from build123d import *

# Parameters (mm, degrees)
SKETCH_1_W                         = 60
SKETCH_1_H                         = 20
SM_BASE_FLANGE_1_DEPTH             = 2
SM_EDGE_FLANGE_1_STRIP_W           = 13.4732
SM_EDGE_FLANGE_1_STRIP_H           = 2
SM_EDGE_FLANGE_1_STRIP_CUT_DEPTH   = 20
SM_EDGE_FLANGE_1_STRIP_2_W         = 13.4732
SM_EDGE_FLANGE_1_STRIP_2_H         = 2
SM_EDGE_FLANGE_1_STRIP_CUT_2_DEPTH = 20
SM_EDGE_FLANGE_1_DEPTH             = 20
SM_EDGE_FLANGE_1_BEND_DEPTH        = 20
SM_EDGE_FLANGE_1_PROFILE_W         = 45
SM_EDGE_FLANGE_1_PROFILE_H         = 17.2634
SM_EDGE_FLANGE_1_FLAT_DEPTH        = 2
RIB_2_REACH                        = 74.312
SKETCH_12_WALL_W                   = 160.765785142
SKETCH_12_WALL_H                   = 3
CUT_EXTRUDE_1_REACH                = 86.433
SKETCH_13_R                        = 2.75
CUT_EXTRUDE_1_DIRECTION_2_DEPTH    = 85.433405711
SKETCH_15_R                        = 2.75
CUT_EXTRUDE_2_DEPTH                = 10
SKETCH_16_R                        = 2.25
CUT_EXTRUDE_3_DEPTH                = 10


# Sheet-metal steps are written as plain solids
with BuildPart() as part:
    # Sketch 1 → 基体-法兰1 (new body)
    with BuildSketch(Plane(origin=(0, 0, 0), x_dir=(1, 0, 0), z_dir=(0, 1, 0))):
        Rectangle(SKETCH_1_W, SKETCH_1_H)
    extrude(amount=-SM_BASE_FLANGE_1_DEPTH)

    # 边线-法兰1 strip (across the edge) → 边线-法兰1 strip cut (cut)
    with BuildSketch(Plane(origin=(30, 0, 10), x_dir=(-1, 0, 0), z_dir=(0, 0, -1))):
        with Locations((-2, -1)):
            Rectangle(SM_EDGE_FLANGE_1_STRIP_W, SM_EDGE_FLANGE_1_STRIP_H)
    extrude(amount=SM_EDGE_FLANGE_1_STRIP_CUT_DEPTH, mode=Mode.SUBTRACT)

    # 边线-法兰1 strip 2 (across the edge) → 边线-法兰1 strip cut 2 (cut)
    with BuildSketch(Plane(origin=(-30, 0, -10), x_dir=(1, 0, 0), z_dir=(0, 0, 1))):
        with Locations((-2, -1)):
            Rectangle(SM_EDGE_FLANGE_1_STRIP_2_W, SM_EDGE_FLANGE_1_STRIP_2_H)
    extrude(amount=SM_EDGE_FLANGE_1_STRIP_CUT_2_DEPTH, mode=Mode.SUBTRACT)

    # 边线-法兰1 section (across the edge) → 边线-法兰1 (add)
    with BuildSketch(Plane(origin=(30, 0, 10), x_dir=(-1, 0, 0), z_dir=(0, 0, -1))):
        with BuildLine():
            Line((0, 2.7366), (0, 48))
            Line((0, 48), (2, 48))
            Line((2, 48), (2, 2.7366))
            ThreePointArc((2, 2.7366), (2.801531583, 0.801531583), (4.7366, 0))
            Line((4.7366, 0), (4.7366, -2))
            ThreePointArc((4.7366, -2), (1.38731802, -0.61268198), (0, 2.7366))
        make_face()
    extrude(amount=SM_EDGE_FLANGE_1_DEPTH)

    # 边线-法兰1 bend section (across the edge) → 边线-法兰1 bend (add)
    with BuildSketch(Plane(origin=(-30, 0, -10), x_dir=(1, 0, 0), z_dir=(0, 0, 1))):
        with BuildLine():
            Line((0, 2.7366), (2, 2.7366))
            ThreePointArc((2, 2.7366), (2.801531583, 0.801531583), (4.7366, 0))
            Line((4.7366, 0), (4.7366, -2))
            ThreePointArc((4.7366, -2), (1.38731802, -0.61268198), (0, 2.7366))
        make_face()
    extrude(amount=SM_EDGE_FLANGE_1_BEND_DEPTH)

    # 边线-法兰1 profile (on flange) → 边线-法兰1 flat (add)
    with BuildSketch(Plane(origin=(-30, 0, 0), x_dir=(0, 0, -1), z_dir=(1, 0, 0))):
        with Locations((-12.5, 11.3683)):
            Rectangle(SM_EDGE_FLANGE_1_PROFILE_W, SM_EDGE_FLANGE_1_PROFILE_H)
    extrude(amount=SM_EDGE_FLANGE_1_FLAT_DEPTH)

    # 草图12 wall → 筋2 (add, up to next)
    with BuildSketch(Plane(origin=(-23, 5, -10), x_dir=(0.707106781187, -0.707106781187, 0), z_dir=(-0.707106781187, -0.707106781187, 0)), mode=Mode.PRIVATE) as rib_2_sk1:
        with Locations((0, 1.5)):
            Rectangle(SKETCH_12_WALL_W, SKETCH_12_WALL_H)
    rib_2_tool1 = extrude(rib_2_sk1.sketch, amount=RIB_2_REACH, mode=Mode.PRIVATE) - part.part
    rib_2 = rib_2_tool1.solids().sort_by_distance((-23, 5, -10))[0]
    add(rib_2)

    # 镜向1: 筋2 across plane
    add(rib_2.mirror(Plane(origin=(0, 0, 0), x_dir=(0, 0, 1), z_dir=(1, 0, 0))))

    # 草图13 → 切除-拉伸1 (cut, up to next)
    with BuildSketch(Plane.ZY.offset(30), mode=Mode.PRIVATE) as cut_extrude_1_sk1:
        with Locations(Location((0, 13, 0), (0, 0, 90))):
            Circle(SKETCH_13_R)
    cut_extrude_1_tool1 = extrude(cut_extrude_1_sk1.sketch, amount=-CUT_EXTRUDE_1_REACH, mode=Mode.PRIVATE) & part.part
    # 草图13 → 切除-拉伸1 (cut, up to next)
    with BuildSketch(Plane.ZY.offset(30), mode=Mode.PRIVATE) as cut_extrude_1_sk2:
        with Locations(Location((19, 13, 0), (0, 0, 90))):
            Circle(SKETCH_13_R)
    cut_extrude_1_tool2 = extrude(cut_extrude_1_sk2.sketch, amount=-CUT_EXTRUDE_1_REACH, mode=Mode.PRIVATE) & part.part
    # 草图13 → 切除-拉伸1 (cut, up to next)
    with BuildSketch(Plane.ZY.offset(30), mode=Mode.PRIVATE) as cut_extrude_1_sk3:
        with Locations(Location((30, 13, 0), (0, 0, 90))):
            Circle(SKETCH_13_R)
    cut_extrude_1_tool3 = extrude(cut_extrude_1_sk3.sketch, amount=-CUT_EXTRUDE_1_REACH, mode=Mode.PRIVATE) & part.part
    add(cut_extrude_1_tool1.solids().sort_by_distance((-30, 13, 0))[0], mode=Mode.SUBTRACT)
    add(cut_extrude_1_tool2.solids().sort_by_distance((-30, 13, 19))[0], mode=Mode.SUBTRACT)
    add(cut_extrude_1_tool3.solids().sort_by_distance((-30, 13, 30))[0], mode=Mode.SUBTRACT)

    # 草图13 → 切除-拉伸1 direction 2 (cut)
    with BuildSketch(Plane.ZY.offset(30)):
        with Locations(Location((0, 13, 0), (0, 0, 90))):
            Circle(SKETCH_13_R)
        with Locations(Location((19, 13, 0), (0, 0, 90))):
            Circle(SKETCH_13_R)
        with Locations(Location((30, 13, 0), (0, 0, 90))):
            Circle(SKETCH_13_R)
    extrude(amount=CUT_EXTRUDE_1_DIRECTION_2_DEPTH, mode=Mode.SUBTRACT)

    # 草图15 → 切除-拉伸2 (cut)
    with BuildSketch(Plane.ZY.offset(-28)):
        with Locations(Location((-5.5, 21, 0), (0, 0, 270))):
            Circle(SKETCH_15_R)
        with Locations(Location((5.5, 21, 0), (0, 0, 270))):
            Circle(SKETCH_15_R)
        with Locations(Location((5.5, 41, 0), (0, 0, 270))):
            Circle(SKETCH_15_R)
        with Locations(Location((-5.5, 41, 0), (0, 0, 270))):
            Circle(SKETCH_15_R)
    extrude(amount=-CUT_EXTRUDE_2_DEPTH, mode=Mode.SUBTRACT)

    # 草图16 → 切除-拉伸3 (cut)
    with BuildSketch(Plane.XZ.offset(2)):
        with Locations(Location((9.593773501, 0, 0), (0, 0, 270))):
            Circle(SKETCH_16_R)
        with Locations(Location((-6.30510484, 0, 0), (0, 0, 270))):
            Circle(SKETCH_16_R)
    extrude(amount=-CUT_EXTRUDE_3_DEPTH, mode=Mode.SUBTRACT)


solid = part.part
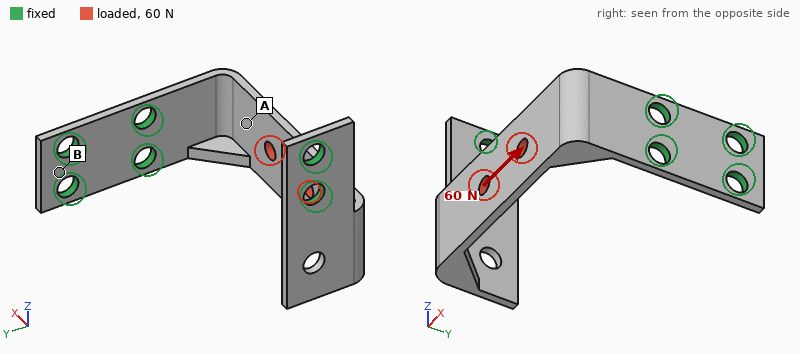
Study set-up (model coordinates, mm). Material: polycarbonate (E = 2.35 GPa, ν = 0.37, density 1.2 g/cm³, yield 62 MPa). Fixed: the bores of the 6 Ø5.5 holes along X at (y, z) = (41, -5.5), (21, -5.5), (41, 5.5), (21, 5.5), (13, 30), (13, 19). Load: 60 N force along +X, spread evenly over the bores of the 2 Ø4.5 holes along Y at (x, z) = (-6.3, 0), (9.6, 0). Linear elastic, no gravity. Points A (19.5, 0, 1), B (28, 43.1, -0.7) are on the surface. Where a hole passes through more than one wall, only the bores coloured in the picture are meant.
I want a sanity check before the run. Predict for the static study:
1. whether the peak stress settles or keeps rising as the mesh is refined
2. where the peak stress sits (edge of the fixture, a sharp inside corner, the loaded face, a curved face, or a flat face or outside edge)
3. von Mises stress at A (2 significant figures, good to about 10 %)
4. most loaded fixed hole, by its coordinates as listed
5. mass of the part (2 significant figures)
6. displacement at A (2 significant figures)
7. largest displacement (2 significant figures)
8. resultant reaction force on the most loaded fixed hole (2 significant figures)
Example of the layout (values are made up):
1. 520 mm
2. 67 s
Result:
1. keeps rising
2. edge of the fixture
3. 8.8 MPa
4. (13, 19)
5. 6.9 g
6. 0.93 mm
7. 1.1 mm
8. 38 N
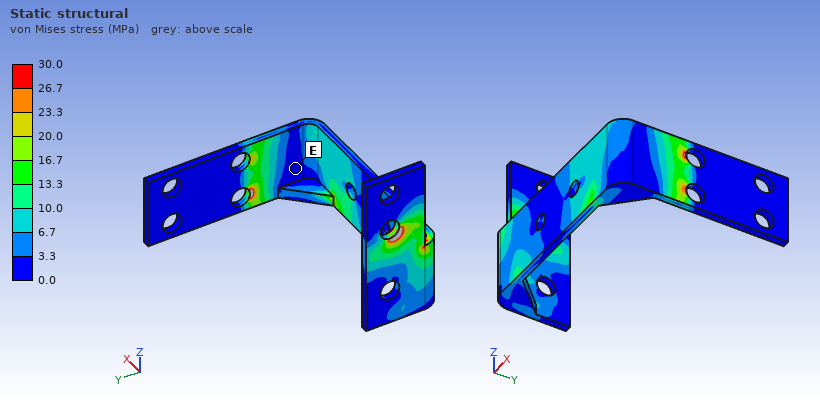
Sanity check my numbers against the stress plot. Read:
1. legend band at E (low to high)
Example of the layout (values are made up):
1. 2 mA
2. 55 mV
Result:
1. 0.0 to 3.3 MPa
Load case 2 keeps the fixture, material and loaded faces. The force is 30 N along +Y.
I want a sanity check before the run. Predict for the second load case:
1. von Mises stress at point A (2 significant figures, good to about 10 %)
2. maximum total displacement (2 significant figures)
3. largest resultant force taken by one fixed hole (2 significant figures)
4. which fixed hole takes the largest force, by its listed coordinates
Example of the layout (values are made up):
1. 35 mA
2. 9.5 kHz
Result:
1. 4.5 MPa
2. 0.94 mm
3. 26 N
4. (13, 19)
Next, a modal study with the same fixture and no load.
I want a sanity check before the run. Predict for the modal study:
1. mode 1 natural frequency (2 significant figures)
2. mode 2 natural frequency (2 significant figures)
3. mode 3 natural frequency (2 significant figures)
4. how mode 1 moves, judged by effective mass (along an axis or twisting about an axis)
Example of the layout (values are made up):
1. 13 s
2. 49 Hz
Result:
1. 640 Hz
2. 830 Hz
3. 1500 Hz
4. along X
